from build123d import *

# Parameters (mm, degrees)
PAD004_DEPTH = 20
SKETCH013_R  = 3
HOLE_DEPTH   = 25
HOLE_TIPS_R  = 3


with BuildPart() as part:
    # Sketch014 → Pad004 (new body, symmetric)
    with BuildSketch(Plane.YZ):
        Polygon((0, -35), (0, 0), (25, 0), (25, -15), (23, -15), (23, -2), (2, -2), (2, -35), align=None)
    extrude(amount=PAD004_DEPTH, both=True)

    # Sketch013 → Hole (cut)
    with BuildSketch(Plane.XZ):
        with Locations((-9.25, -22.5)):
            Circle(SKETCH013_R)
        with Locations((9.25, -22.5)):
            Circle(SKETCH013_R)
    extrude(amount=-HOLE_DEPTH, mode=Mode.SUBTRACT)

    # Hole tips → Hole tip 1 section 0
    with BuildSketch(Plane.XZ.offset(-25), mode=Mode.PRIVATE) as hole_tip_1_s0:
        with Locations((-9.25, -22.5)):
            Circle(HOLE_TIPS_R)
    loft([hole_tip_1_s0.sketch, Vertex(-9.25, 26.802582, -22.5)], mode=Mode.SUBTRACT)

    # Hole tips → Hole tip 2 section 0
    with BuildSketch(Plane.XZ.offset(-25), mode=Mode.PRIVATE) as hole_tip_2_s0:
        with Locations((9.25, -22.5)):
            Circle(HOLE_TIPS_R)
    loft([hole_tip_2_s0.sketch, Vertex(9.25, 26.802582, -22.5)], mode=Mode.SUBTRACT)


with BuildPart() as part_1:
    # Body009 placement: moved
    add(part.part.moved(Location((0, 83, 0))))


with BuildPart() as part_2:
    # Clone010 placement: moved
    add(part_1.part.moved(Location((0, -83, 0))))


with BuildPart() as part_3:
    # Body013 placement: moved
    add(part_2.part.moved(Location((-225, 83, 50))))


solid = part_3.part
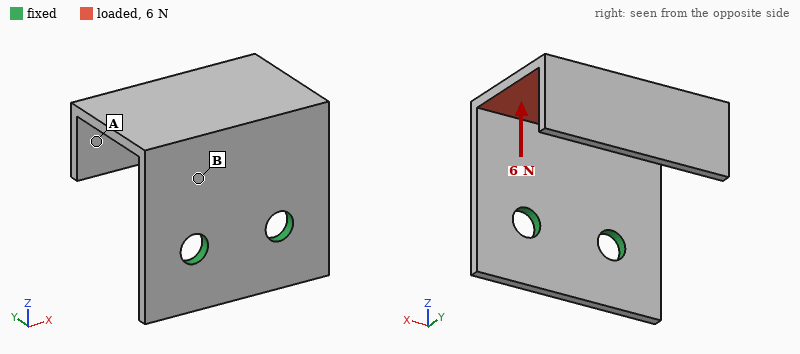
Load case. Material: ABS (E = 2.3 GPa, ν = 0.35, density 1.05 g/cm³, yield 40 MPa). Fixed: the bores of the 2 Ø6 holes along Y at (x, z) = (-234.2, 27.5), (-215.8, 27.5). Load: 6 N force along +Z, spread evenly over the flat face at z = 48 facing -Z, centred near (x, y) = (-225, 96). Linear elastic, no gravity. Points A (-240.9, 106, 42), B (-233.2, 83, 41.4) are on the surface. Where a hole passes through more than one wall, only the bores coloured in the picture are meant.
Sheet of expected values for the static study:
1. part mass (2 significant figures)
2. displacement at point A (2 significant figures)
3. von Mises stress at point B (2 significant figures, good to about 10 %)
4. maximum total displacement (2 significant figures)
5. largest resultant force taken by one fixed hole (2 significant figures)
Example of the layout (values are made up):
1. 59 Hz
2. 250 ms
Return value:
1. 5.8 g
2. 0.55 mm
3. 2.2 MPa
4. 0.65 mm
5. 3.1 N
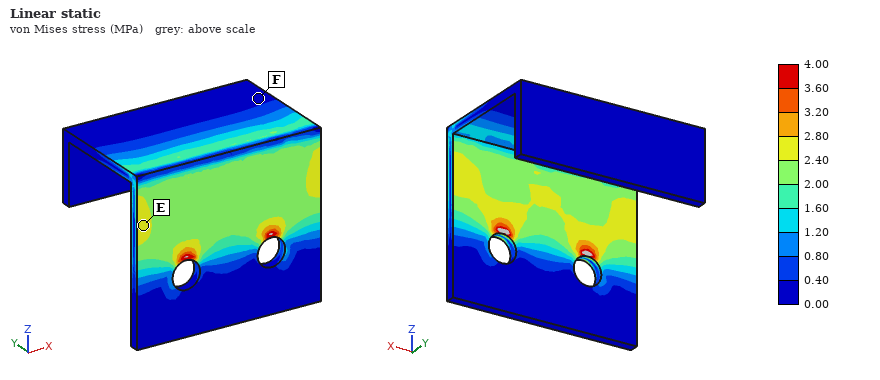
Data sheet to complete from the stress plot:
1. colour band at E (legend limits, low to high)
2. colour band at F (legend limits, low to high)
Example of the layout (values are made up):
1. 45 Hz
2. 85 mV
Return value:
1. 2.40 to 2.80 MPa
2. 0.00 to 0.40 MPa
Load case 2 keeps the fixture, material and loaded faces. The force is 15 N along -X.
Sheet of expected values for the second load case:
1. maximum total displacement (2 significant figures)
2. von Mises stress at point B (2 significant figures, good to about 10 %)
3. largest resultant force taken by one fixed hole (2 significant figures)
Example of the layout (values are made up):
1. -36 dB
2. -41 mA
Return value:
1. 0.62 mm
2. 2.6 MPa
3. 16 N
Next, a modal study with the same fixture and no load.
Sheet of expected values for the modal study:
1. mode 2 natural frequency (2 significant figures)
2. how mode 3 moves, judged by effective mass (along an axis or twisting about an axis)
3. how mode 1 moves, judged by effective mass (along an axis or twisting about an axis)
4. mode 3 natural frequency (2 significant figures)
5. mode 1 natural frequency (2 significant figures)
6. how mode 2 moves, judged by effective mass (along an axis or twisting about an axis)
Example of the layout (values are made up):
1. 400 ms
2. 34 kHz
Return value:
1. 390 Hz
2. along Y
3. along Z
4. 600 Hz
5. 240 Hz
6. along X
